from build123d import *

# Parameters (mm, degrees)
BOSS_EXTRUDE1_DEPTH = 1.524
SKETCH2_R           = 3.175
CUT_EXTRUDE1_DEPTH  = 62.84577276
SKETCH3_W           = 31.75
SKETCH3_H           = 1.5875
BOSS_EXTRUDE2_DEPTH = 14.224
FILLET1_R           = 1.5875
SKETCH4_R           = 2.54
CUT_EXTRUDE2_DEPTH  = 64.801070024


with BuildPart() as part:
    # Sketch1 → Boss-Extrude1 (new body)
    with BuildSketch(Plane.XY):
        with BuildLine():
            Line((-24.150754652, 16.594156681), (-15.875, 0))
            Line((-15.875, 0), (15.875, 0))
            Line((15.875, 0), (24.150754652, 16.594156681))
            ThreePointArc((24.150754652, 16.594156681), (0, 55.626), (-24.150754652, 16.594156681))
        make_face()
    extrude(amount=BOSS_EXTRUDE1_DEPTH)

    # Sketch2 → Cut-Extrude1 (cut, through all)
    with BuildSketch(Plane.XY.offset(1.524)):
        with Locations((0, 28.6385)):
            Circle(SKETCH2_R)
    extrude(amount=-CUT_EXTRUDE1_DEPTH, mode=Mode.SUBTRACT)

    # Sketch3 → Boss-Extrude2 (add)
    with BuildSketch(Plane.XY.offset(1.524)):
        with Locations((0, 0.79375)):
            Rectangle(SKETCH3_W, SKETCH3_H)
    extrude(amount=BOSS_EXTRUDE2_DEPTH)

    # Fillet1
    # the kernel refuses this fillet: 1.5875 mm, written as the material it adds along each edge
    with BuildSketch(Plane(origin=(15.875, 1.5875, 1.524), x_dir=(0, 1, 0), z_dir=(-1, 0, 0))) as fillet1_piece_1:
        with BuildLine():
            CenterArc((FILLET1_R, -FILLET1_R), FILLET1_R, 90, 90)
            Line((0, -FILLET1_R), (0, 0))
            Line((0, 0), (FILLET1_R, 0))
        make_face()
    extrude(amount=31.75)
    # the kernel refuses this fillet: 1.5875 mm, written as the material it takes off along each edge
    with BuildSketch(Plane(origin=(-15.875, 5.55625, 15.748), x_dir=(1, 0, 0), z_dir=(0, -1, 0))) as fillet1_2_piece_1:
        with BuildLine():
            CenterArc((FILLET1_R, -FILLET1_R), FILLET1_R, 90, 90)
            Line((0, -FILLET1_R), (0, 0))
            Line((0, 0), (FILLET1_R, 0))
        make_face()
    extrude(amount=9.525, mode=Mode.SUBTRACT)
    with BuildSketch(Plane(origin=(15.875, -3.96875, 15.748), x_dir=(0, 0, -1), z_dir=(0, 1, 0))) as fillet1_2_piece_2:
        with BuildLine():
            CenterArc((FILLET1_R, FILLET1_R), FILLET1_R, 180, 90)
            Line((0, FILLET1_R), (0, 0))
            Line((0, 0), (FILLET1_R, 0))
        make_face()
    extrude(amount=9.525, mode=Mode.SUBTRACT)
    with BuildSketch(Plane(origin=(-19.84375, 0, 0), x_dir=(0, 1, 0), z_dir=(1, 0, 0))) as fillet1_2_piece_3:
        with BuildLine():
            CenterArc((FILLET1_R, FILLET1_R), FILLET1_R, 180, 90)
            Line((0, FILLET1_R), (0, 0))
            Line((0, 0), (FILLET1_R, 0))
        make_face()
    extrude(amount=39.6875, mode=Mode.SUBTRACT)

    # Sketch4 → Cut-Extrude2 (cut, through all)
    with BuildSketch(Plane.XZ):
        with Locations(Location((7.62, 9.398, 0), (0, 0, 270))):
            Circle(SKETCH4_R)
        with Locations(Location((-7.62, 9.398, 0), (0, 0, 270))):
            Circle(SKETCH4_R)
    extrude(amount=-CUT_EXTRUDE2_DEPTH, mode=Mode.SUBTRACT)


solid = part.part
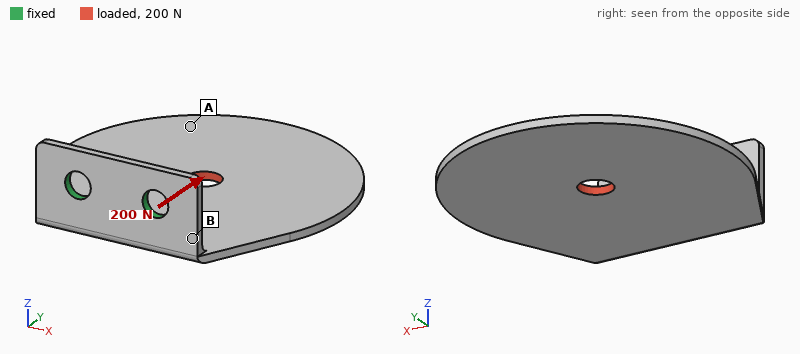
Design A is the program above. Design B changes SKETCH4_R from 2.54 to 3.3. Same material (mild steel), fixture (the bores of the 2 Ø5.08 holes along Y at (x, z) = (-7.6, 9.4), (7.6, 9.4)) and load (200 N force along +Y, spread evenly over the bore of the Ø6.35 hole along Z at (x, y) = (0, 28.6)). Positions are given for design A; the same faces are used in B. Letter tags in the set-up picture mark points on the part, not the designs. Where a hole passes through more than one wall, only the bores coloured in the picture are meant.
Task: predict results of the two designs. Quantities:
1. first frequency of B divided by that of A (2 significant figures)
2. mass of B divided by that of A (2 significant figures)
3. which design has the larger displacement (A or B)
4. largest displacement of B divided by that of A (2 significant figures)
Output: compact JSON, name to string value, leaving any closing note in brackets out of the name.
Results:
{"first frequency of B divided by that of A": "1.0", "mass of B divided by that of A": "0.99", "which design has the larger displacement": "A", "largest displacement of B divided by that of A": "0.77"}
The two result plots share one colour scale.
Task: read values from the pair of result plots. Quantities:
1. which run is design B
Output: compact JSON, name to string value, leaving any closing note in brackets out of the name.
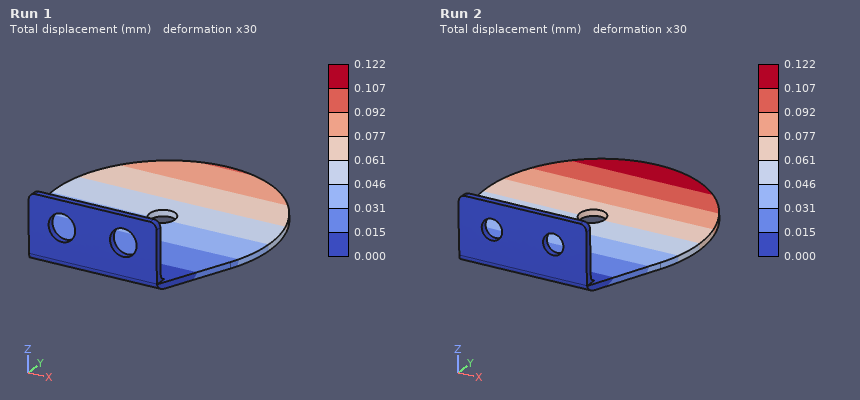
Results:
{"which run is design B": "Run 1"}
